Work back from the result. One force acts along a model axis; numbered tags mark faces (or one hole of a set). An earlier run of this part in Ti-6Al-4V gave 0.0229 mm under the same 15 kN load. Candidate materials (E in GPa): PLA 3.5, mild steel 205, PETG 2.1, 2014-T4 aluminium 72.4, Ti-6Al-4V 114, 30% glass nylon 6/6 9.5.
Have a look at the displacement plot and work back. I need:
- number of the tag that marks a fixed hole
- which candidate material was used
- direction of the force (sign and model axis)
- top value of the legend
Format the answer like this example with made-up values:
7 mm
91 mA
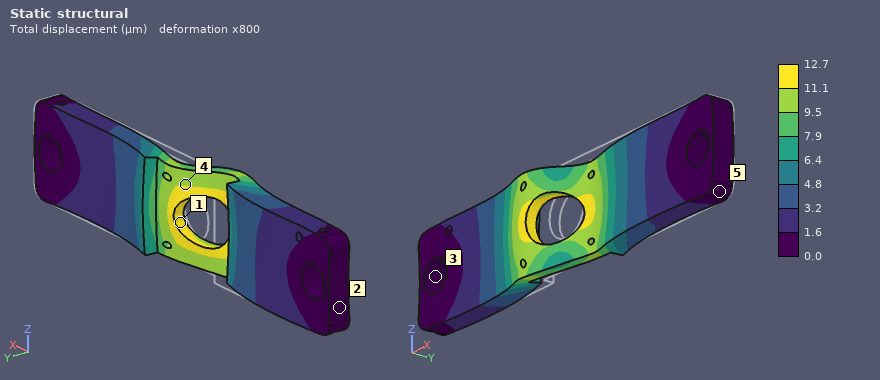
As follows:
3
mild steel
-X
12.7 µm
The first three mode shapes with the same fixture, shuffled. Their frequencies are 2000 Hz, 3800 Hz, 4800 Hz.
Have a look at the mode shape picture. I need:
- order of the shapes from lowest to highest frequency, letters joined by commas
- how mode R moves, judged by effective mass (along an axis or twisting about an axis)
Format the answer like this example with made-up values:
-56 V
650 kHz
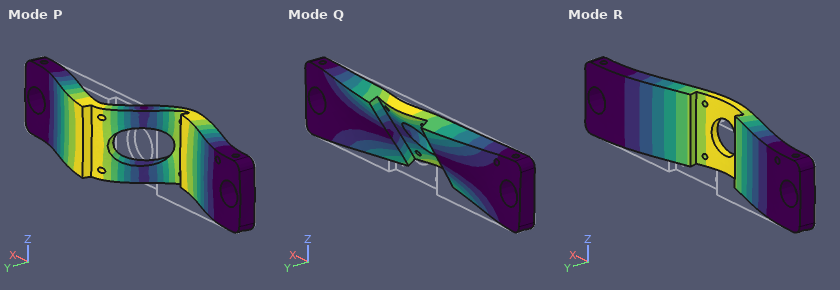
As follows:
R, P, Q
along Y
